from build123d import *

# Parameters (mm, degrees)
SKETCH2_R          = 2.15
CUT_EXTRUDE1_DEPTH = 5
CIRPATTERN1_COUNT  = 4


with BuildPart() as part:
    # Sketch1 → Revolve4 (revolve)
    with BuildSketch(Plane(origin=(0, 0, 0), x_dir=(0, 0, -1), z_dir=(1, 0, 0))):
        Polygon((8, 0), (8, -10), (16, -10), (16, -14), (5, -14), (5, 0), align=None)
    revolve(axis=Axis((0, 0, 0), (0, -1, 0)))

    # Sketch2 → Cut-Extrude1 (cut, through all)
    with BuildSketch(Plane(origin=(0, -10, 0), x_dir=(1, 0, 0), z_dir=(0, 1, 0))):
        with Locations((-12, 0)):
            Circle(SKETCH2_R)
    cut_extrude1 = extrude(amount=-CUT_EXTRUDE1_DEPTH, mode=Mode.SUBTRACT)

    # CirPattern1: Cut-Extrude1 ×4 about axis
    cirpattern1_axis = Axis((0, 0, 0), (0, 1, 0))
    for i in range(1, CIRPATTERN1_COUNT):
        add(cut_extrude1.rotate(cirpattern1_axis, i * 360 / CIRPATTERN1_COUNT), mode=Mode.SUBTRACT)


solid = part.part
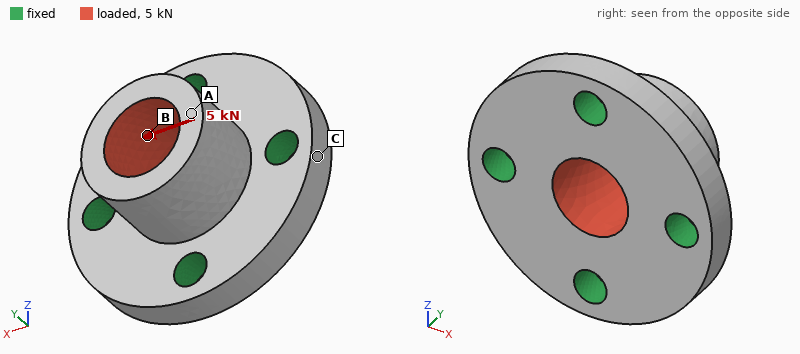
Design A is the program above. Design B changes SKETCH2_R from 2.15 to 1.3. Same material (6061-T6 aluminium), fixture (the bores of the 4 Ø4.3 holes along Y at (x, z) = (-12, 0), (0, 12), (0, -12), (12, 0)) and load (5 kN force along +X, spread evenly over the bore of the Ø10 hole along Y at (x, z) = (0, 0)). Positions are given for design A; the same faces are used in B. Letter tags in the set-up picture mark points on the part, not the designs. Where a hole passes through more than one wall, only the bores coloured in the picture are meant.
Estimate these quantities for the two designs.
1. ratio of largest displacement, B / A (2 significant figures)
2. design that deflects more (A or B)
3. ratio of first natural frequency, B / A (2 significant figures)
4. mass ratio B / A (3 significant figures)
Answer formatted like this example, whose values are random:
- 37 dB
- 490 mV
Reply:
- 1.2
- B
- 0.88
- 1.04
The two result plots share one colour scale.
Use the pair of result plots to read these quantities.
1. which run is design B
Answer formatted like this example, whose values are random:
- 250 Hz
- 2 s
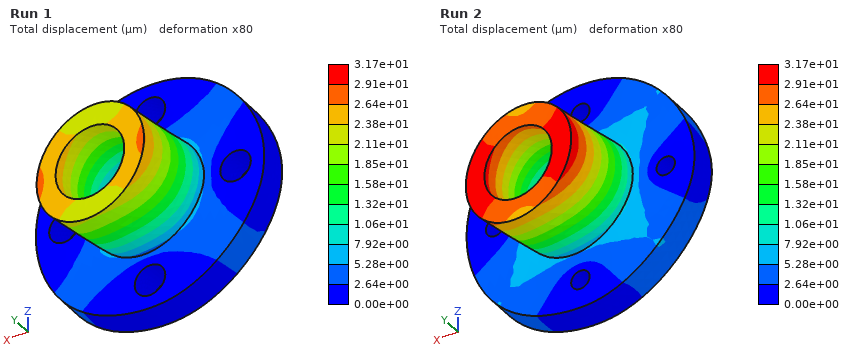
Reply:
- Run 2
